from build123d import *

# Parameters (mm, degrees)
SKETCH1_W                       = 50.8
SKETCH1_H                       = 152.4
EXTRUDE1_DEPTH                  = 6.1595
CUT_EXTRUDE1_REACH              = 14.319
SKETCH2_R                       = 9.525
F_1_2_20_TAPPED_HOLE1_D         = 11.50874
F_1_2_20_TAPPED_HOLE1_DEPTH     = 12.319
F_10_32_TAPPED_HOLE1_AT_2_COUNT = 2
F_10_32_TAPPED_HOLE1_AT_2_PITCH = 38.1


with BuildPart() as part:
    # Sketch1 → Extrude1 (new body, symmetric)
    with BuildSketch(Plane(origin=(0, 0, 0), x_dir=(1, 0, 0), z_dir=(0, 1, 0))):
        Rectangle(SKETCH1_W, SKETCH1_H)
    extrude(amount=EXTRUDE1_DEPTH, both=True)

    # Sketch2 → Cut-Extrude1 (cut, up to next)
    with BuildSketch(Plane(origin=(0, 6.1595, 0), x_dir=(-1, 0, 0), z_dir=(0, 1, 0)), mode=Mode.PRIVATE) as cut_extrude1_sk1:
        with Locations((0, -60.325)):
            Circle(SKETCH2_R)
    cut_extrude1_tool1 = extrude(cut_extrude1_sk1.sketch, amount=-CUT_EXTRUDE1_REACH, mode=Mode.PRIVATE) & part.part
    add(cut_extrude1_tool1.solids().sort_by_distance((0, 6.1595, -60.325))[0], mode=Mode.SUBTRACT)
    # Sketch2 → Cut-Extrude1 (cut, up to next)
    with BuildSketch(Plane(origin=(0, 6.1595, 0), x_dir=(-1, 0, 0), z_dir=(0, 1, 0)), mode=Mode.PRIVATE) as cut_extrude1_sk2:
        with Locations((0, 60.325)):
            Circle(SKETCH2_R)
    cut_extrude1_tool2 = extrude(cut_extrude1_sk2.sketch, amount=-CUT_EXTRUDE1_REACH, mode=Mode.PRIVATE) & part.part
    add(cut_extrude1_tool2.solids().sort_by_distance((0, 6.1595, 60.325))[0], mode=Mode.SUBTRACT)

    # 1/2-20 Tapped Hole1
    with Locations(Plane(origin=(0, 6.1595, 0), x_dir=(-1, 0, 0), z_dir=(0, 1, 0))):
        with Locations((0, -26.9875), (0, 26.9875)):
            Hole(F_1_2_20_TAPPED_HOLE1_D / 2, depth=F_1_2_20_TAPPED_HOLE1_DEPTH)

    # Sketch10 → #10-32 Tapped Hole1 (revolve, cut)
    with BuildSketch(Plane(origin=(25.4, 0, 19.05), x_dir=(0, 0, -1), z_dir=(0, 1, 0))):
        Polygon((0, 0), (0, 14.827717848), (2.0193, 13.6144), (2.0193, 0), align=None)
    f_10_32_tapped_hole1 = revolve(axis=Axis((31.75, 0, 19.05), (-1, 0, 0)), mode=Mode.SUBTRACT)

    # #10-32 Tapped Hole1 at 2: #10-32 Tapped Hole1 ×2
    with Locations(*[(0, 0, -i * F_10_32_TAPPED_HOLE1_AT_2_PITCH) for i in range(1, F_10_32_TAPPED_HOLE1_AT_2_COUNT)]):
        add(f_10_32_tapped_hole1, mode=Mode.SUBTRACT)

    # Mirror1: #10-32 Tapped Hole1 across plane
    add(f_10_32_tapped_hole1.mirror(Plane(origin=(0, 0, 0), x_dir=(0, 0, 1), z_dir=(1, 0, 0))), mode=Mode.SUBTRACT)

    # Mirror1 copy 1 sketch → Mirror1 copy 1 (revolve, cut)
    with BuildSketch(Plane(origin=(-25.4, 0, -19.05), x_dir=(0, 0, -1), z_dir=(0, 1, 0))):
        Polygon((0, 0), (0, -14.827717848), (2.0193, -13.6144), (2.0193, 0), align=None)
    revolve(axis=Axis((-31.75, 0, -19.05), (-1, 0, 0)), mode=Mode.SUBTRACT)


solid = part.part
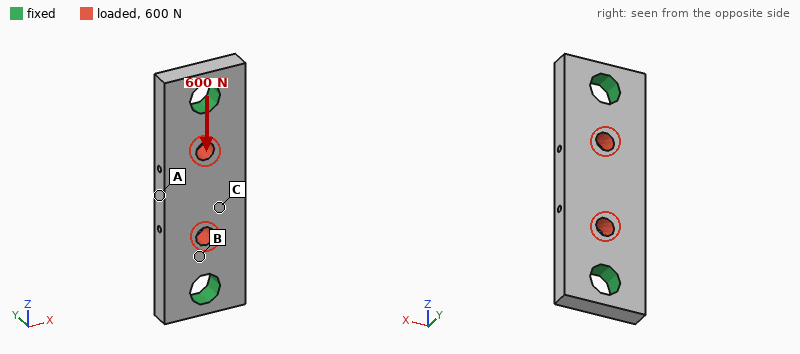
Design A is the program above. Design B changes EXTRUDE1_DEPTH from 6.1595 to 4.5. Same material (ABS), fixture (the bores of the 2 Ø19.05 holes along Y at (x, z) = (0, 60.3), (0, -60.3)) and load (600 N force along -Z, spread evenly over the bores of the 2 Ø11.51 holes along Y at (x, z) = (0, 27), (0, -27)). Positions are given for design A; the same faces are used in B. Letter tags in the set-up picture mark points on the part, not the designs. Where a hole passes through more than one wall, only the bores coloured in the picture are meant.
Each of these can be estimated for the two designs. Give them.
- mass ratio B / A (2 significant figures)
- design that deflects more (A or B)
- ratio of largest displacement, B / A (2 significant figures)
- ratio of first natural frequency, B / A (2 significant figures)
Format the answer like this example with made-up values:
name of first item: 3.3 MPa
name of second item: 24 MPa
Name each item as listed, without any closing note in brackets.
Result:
mass ratio B / A: 0.73
design that deflects more: B
ratio of largest displacement, B / A: 1.4
ratio of first natural frequency, B / A: 0.77
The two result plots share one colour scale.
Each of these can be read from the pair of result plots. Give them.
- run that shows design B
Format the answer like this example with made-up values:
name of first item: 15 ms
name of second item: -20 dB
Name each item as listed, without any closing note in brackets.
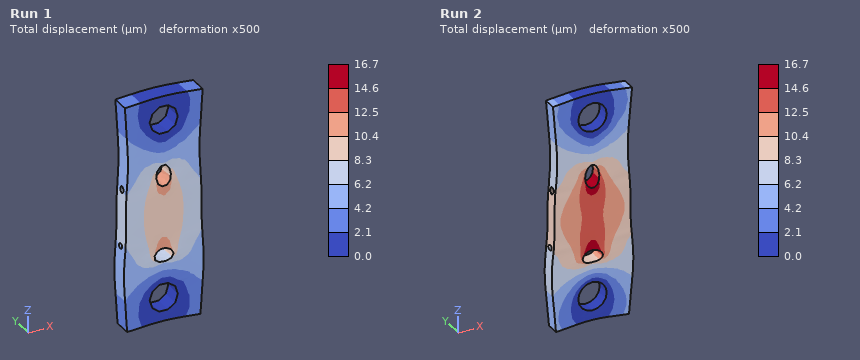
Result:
run that shows design B: Run 2
